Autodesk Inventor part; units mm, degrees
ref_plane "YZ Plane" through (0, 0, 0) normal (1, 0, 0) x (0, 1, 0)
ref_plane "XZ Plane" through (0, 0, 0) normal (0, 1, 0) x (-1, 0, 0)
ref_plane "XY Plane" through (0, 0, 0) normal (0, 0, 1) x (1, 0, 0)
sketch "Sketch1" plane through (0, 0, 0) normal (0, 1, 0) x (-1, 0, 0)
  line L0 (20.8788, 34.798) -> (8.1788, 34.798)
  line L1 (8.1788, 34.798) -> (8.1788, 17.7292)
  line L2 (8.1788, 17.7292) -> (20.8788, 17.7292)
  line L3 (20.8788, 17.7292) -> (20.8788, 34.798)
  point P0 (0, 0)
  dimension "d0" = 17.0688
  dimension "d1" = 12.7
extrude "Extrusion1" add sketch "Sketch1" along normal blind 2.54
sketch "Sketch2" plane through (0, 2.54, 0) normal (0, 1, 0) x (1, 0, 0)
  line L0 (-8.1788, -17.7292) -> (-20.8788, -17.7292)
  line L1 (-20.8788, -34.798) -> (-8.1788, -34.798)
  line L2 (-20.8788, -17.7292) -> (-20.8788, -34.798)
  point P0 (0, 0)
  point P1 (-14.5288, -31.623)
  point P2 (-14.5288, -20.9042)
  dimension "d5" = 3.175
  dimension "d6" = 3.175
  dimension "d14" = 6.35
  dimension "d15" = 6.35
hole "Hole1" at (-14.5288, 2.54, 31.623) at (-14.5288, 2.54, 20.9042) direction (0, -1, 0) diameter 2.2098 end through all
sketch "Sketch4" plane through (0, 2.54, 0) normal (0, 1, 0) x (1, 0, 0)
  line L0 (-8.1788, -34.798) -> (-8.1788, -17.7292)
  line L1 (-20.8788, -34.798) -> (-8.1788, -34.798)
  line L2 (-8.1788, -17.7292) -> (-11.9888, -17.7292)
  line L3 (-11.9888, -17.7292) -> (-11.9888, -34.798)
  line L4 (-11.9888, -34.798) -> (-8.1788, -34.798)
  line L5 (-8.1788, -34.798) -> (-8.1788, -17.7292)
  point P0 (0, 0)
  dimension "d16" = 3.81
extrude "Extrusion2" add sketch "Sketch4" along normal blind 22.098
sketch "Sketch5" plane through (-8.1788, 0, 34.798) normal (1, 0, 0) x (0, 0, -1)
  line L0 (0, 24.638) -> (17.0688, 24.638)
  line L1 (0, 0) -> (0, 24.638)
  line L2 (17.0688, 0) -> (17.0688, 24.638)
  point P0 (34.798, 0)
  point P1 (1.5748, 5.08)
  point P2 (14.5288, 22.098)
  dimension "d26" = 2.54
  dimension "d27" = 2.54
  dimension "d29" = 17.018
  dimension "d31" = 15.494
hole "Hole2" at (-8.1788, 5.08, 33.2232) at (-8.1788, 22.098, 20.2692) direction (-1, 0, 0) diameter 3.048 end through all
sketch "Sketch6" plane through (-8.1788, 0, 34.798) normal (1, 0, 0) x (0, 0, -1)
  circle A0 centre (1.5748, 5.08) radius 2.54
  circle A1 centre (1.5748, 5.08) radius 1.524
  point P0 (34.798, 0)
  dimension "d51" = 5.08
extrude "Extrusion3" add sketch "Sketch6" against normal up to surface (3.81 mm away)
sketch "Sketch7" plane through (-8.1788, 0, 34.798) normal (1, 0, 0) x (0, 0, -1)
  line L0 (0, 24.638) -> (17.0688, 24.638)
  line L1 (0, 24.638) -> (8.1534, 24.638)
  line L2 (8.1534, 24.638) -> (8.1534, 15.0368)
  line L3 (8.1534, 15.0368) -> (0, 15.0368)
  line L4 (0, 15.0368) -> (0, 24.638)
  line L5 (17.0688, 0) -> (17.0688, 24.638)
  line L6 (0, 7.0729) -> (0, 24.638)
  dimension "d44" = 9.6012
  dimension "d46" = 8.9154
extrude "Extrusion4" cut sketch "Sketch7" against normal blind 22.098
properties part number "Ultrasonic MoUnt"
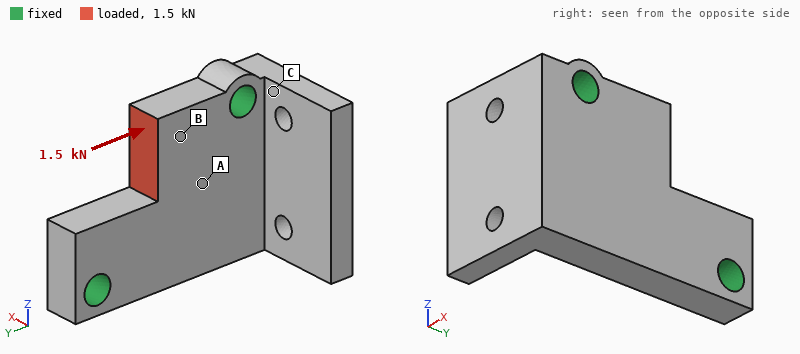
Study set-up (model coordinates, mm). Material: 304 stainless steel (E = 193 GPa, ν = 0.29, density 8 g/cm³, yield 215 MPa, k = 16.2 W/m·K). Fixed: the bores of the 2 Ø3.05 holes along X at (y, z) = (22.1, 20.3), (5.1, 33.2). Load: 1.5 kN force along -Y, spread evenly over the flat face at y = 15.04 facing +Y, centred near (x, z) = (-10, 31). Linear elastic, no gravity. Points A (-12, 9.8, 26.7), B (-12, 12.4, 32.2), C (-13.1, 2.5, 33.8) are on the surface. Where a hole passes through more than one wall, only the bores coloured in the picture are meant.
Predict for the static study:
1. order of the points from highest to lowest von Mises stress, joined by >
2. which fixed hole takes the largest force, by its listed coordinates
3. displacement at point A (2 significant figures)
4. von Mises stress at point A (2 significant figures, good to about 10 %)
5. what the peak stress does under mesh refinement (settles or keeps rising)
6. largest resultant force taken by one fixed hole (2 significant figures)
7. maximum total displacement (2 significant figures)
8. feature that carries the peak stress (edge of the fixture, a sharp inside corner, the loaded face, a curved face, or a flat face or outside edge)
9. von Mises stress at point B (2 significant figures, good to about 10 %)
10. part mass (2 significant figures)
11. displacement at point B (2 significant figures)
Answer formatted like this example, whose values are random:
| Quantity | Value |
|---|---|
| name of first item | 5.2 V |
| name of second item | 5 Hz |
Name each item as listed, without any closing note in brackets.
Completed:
| Quantity | Value |
|---|---|
| order of the points from highest to lowest von Mises stress, joined by > | B > A > C |
| which fixed hole takes the largest force, by its listed coordinates | (5.1, 33.2) |
| displacement at point A | 1.2 µm |
| von Mises stress at point A | 16 MPa |
| what the peak stress does under mesh refinement | keeps rising |
| largest resultant force taken by one fixed hole | 1.1 kN |
| maximum total displacement | 2.5 µm |
| feature that carries the peak stress | edge of the fixture |
| von Mises stress at point B | 50 MPa |
| part mass | 13 g |
| displacement at point B | 1.7 µm |
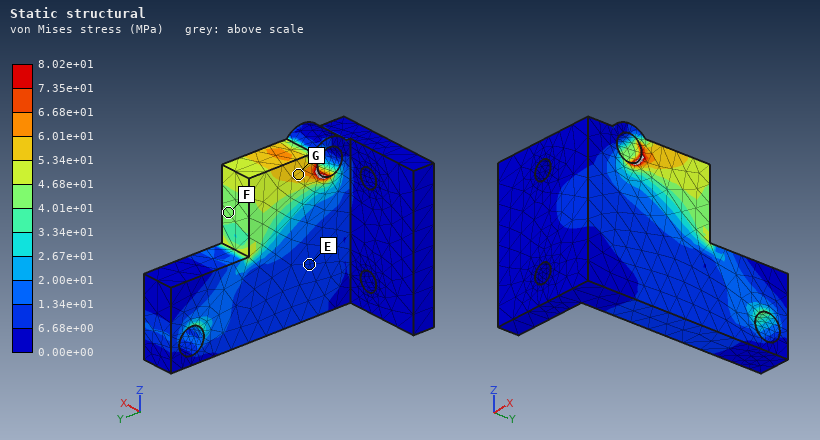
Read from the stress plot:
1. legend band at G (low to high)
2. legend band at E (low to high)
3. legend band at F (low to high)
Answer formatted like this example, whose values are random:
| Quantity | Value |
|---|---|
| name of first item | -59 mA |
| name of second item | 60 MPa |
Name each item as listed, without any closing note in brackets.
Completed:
| Quantity | Value |
|---|---|
| legend band at G | 5.34e+01 to 6.01e+01 MPa |
| legend band at E | 6.68e+00 to 1.34e+01 MPa |
| legend band at F | 4.01e+01 to 4.68e+01 MPa |
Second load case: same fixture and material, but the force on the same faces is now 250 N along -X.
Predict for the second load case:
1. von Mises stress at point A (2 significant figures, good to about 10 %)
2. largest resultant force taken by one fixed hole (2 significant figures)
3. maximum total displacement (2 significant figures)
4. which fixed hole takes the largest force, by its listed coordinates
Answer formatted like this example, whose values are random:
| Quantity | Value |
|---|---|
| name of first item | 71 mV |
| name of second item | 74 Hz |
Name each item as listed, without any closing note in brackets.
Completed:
| Quantity | Value |
|---|---|
| von Mises stress at point A | 23 MPa |
| largest resultant force taken by one fixed hole | 160 N |
| maximum total displacement | 6.7 µm |
| which fixed hole takes the largest force, by its listed coordinates | (5.1, 33.2) |
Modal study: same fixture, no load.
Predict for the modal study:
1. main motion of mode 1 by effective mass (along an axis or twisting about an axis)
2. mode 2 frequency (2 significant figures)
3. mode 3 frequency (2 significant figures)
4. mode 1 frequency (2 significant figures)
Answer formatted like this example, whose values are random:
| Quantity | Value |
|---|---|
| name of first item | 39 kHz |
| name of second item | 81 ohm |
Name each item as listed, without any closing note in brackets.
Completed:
| Quantity | Value |
|---|---|
| main motion of mode 1 by effective mass | along X |
| mode 2 frequency | 16 kHz |
| mode 3 frequency | 27 kHz |
| mode 1 frequency | 11 kHz |
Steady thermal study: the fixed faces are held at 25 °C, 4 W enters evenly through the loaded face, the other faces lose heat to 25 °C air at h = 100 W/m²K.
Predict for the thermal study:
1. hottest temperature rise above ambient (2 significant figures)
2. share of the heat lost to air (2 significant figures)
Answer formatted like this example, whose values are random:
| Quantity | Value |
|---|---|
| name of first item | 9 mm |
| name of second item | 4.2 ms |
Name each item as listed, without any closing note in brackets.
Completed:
| Quantity | Value |
|---|---|
| hottest temperature rise above ambient | 53 K |
| share of the heat lost to air | 26 % |
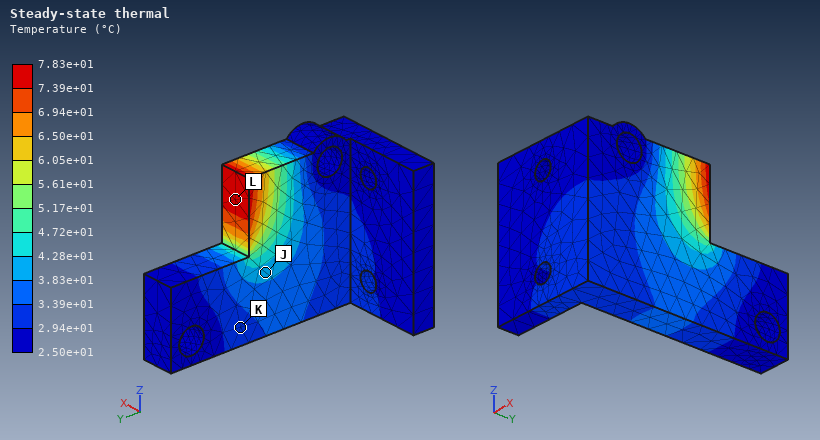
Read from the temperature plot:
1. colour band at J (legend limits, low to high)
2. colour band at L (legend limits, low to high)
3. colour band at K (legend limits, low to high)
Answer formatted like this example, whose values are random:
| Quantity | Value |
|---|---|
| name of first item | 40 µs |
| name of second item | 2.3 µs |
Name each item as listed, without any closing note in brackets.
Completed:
| Quantity | Value |
|---|---|
| colour band at J | 3.83e+01 to 4.28e+01 °C |
| colour band at L | 7.39e+01 to 7.83e+01 °C |
| colour band at K | 2.94e+01 to 3.39e+01 °C |
